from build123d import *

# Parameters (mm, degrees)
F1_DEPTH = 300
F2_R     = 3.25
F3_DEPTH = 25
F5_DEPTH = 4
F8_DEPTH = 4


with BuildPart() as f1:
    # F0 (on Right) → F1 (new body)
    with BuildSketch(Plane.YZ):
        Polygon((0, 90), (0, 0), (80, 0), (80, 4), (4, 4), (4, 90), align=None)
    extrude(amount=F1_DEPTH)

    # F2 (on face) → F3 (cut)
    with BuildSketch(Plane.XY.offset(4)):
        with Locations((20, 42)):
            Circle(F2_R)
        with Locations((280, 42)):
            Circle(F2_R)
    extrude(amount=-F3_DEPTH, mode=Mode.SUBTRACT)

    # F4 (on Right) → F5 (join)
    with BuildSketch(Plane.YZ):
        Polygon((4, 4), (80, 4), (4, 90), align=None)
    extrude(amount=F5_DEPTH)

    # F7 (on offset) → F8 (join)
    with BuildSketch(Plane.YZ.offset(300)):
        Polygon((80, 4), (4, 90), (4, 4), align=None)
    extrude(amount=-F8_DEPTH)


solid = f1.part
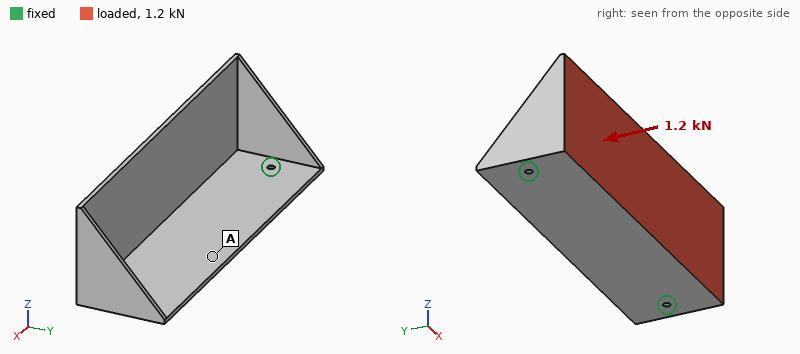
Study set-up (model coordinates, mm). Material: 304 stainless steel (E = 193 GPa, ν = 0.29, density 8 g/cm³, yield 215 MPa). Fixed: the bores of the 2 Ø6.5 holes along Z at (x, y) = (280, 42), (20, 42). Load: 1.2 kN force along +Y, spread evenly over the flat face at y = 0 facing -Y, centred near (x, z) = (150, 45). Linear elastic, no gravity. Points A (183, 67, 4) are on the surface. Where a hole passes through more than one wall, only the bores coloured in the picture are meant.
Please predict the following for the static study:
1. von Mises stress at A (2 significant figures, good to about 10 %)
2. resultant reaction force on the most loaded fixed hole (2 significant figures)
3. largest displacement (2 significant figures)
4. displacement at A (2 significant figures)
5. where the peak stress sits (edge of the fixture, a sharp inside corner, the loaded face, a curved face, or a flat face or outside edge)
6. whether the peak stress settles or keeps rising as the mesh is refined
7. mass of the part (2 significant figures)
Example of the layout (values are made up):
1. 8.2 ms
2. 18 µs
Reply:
1. 12 MPa
2. 650 N
3. 0.75 mm
4. 0.21 mm
5. edge of the fixture
6. keeps rising
7. 1.8 kg
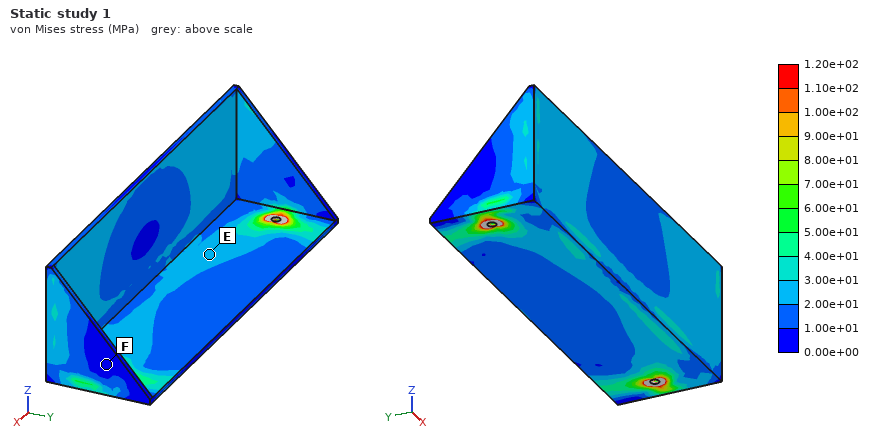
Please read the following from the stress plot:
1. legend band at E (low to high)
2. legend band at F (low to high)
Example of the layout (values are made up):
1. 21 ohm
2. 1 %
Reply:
1. 2.00e+01 to 3.00e+01 MPa
2. 0.00e+00 to 1.00e+01 MPa
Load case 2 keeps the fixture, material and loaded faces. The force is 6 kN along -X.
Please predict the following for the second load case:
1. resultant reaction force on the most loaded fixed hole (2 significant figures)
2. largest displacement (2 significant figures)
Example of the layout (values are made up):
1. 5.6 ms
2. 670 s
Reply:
1. 3.3 kN
2. 0.41 mm
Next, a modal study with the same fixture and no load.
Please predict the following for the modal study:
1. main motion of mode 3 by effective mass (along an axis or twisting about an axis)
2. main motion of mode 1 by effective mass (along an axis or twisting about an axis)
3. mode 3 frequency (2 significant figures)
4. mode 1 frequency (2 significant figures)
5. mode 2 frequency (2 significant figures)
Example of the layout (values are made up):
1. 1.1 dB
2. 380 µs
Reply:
1. along Z
2. along Y
3. 460 Hz
4. 260 Hz
5. 430 Hz
